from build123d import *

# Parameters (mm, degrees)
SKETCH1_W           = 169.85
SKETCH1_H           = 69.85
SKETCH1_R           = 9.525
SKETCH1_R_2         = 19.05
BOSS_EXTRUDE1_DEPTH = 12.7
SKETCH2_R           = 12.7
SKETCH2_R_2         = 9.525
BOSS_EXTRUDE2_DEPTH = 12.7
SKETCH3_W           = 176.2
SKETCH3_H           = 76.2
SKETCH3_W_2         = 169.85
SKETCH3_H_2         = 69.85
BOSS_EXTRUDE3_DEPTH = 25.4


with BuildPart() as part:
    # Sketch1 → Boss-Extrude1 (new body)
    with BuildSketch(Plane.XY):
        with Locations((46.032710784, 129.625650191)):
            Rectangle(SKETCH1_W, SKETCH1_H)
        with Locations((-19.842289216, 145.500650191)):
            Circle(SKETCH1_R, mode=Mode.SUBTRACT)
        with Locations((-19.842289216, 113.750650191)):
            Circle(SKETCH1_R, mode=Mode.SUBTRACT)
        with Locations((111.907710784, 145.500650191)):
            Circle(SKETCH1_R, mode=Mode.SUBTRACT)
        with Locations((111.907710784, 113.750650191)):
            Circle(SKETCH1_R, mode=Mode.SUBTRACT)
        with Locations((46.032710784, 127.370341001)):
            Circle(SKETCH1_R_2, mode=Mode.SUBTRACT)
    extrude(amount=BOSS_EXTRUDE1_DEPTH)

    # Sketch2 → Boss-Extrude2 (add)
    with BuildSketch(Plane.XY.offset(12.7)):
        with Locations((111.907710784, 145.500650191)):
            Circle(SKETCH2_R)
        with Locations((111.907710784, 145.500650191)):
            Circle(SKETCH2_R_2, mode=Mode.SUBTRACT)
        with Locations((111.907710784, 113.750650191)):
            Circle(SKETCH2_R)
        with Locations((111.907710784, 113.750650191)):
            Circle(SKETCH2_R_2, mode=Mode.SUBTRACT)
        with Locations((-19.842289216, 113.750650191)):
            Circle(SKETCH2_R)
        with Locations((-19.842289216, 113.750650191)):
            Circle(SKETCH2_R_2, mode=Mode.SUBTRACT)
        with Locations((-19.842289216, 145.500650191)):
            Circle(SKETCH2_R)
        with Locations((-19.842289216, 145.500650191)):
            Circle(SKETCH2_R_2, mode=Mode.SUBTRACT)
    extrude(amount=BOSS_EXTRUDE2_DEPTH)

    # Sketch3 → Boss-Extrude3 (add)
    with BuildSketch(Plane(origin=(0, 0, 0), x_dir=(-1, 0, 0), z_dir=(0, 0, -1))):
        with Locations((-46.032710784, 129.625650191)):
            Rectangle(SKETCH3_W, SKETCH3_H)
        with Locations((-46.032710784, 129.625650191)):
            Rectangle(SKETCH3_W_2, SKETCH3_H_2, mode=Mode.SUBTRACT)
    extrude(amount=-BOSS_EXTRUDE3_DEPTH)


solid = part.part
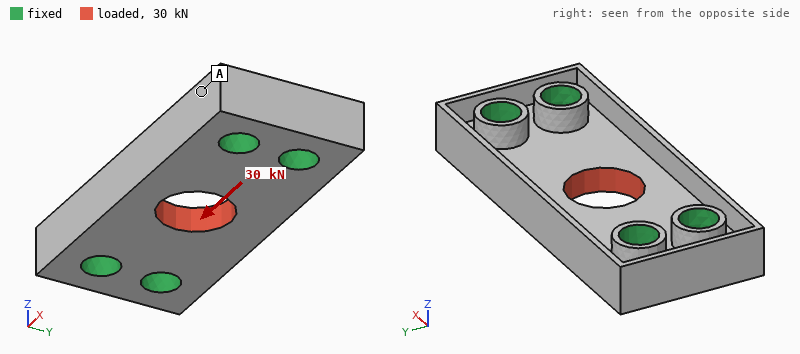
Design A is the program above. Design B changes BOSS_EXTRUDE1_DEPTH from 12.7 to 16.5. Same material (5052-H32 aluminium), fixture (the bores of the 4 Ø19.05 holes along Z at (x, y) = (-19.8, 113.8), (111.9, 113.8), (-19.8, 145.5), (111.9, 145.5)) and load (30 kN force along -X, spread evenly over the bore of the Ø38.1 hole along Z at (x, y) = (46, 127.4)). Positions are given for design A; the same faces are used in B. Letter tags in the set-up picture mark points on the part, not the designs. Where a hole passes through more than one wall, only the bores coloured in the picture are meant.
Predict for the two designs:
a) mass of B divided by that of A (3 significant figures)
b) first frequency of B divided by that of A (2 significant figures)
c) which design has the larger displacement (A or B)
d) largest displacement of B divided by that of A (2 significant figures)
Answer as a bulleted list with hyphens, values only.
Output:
- 1.19
- 1.1
- A
- 0.77
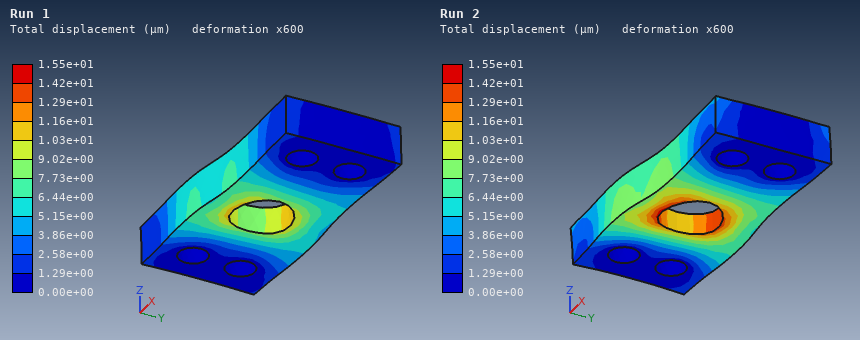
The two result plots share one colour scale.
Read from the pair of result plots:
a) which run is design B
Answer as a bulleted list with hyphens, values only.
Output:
- Run 1
